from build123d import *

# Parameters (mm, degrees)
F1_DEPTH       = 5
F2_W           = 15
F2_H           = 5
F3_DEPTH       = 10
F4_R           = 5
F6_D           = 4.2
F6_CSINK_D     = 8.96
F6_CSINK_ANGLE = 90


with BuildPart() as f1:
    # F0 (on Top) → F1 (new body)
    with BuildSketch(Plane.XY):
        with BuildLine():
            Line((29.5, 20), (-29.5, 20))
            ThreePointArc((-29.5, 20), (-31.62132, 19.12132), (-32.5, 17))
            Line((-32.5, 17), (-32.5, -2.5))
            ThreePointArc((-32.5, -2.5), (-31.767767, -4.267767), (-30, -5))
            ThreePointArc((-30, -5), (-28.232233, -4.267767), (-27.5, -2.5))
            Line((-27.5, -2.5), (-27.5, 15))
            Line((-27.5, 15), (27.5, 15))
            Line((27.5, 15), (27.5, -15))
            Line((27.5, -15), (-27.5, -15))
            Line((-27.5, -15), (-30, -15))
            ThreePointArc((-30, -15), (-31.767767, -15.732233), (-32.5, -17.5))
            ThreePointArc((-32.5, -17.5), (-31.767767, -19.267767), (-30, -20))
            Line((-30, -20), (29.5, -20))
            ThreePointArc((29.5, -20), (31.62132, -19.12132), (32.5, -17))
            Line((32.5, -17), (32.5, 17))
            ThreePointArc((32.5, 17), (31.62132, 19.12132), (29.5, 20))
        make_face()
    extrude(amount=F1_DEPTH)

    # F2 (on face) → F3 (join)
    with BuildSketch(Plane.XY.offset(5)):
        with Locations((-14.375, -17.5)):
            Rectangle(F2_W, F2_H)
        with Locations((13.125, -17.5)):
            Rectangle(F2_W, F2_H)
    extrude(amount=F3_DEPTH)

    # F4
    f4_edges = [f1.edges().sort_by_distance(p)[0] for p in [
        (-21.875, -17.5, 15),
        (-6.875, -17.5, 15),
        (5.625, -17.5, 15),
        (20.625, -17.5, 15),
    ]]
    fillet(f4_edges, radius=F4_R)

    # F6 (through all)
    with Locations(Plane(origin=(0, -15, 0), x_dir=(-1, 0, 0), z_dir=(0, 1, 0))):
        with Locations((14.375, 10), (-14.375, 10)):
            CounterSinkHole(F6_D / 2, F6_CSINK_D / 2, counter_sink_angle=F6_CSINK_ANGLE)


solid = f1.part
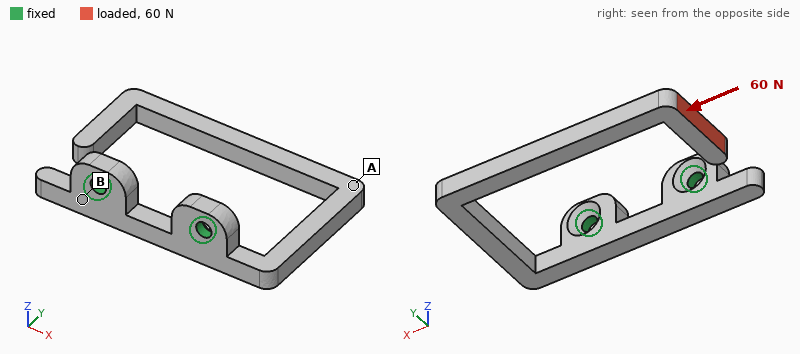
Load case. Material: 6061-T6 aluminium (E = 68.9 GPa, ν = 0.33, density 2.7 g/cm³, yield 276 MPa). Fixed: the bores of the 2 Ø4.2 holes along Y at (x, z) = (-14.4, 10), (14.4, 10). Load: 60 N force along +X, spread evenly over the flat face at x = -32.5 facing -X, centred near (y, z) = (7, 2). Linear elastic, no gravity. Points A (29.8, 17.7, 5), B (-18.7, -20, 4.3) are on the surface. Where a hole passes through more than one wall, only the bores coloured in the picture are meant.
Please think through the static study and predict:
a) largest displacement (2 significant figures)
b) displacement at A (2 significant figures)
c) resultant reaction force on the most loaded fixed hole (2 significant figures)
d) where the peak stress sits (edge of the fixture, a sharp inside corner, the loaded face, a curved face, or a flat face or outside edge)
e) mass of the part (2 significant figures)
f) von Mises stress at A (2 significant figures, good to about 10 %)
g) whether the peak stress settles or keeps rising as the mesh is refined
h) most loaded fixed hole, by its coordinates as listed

0.44 mm
0.35 mm
43 N
edge of the fixture
15 g
15 MPa
keeps rising
(-14.4, 10)
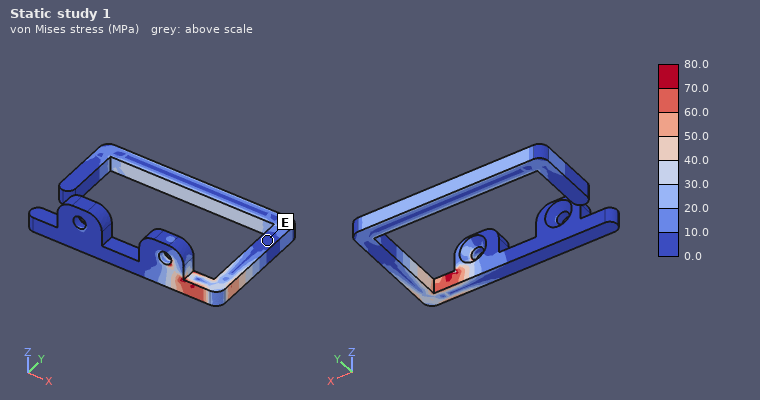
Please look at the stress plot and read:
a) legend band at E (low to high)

0.0 to 10.0 MPa
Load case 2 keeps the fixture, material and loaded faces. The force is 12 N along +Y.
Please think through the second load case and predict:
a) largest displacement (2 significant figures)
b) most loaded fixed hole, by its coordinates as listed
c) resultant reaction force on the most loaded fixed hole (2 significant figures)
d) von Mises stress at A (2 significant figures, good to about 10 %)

0.87 mm
(-14.4, 10)
10 N
21 MPa
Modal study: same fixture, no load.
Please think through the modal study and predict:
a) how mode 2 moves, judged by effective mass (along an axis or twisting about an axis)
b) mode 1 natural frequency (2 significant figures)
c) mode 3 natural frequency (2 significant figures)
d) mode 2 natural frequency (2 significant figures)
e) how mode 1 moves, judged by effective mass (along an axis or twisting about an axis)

along Y
320 Hz
990 Hz
360 Hz
along Z
